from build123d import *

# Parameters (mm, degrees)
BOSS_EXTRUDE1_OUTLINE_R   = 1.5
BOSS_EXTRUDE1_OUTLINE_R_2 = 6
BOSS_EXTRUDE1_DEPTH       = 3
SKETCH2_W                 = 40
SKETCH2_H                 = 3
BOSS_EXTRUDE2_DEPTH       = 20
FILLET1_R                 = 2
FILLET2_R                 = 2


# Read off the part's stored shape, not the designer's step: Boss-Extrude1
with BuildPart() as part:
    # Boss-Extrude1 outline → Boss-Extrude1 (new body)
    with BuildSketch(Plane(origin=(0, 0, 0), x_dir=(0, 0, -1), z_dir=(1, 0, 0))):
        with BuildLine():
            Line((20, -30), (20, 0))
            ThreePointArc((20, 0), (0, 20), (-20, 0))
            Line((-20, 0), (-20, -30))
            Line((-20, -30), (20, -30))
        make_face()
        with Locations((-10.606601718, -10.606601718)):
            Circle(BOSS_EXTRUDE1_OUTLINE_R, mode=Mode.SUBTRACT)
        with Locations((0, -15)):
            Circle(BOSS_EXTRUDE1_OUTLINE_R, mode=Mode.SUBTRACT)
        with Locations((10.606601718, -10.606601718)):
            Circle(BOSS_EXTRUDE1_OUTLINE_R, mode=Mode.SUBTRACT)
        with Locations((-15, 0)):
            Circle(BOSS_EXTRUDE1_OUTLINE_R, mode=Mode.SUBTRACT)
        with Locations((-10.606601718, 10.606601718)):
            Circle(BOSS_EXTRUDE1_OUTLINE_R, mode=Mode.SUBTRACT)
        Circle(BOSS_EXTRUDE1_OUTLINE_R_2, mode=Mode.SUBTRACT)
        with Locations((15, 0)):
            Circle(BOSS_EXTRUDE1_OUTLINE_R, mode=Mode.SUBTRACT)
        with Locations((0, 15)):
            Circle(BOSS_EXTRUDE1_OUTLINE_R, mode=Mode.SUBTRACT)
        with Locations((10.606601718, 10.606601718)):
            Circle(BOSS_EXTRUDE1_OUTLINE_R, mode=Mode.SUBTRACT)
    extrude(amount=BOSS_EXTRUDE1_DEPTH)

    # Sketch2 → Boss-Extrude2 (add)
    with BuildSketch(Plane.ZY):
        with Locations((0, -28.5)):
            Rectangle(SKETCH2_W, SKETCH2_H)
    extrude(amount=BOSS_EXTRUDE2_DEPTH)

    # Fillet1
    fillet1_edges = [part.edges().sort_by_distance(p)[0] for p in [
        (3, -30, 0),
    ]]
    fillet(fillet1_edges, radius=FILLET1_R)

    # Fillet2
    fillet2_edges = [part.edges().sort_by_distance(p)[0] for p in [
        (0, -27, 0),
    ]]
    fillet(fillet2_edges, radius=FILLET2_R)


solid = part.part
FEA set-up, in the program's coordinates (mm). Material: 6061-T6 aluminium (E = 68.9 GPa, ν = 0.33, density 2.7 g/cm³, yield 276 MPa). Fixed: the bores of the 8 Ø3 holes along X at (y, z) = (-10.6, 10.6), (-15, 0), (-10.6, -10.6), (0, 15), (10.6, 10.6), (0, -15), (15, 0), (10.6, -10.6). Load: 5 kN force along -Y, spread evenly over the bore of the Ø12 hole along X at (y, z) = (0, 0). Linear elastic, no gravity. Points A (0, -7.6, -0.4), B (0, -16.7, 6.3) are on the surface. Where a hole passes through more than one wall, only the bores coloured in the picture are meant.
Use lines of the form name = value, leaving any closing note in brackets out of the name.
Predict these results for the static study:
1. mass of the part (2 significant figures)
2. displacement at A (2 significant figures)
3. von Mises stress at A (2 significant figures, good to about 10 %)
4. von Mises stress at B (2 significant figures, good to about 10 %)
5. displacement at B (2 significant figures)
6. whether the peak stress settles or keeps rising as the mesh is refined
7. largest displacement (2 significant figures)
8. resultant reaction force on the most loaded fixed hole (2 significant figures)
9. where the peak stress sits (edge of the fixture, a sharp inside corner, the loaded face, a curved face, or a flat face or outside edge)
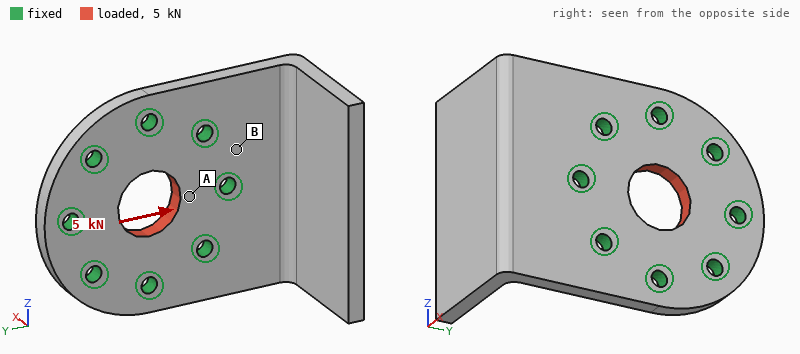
mass of the part = 20 g
displacement at A = 4.3 µm
von Mises stress at A = 43 MPa
von Mises stress at B = 9.9 MPa
displacement at B = 1.0 µm
whether the peak stress settles or keeps rising as the mesh is refined = keeps rising
largest displacement = 5.9 µm
resultant reaction force on the most loaded fixed hole = 1.0 kN
where the peak stress sits = edge of the fixture
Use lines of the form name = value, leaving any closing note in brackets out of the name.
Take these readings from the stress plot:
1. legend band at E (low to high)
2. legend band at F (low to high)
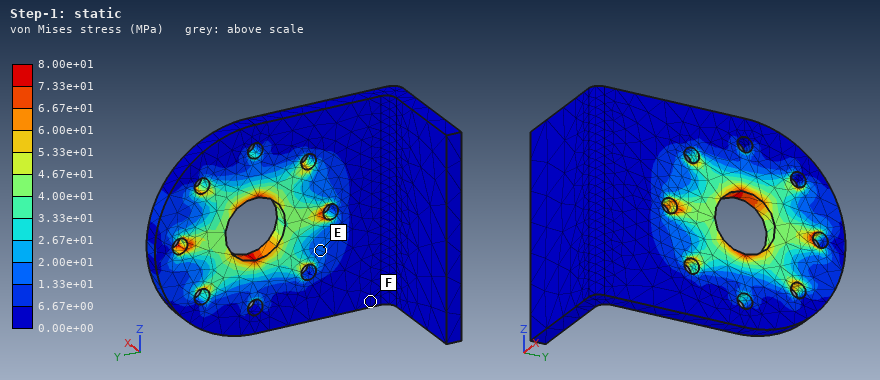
legend band at E = 1.33e+01 to 2.00e+01 MPa
legend band at F = 0.00e+00 to 6.67e+00 MPa
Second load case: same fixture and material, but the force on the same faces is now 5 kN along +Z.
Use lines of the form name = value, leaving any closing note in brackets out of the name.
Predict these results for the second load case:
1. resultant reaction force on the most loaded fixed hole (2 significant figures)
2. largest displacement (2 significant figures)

resultant reaction force on the most loaded fixed hole = 1.0 kN
largest displacement = 5.9 µm
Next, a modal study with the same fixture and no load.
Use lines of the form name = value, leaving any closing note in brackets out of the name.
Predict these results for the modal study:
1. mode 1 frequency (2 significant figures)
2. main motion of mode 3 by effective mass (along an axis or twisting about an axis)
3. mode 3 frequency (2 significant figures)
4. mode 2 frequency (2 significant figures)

mode 1 frequency = 2500 Hz
main motion of mode 3 by effective mass = along X
mode 3 frequency = 7300 Hz
mode 2 frequency = 3800 Hz
